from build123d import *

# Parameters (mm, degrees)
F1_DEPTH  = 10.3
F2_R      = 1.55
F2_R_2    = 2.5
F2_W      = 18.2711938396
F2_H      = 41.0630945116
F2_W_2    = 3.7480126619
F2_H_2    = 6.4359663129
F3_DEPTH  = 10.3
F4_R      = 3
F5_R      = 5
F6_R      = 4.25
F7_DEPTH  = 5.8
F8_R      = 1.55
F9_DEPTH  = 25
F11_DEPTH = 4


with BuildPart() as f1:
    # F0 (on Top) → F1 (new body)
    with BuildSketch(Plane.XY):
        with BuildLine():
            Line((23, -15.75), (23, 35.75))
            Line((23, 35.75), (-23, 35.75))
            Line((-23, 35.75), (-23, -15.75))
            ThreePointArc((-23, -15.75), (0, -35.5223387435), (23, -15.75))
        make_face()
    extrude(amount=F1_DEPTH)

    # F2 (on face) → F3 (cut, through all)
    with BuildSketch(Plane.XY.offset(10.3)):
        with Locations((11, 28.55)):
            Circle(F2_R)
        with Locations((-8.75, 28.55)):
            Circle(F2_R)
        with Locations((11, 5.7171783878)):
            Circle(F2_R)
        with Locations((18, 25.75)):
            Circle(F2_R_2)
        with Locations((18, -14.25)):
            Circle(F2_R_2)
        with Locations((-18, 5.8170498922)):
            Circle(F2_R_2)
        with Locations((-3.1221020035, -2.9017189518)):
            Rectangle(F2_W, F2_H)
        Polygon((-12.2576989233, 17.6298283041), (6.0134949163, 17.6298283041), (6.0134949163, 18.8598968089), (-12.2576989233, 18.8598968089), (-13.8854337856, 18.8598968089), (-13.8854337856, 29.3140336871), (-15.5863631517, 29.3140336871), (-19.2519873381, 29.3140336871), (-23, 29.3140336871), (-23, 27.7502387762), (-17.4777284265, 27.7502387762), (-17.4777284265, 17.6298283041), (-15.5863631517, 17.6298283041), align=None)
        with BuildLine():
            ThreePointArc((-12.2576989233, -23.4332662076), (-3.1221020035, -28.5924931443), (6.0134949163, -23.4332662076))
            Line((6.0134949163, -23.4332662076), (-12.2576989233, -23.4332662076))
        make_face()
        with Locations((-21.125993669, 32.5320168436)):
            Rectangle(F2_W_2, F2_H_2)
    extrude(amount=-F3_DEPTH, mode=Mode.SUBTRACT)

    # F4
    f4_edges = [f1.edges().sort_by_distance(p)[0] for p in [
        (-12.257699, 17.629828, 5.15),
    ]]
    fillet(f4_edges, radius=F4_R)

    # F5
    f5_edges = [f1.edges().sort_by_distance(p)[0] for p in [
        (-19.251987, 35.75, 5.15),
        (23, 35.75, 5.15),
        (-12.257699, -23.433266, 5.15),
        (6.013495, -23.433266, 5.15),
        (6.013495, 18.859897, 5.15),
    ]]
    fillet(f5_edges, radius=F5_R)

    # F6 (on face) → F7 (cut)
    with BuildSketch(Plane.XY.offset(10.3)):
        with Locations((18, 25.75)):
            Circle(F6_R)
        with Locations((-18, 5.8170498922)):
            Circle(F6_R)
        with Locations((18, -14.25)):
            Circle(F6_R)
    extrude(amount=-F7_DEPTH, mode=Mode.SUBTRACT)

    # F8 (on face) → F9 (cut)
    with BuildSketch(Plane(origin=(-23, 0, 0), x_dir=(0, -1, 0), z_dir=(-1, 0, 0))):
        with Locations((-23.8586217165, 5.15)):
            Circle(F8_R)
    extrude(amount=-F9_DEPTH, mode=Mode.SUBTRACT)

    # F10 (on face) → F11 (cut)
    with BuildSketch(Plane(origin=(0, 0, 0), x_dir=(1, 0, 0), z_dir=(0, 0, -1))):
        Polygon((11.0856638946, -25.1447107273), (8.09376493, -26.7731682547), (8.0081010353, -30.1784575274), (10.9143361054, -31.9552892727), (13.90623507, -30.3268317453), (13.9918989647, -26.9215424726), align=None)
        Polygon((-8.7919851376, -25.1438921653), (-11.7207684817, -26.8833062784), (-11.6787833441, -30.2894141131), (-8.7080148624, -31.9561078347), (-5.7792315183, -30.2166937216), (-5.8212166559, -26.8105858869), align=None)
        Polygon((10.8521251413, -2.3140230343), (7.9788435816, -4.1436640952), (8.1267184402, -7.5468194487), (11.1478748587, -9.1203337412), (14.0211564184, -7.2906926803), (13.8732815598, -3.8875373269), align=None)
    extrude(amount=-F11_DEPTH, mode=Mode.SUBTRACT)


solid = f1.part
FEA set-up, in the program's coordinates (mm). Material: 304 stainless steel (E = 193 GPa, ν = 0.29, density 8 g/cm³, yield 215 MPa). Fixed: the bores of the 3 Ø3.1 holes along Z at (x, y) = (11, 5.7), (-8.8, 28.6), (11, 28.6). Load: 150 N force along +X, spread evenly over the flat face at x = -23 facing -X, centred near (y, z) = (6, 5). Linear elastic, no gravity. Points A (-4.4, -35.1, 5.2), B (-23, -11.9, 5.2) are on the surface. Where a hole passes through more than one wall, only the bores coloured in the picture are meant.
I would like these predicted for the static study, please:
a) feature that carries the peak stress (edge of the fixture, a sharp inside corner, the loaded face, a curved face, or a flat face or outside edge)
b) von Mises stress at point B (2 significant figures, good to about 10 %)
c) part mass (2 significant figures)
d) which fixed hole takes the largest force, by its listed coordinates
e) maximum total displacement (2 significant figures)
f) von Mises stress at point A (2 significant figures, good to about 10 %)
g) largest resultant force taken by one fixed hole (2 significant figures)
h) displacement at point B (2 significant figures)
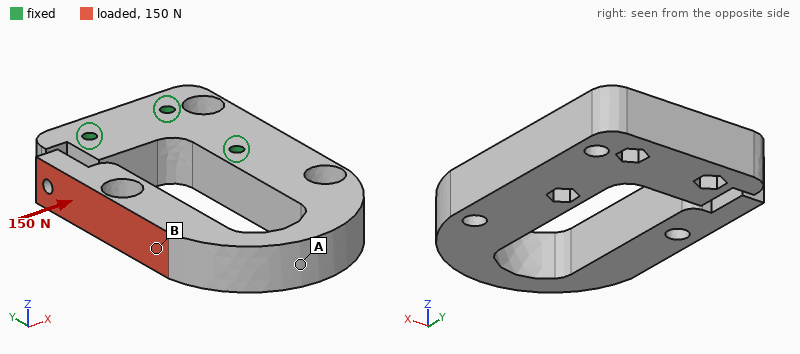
a curved face
13 MPa
160 g
(11, 5.7)
0.20 mm
64 MPa
140 N
0.079 mm
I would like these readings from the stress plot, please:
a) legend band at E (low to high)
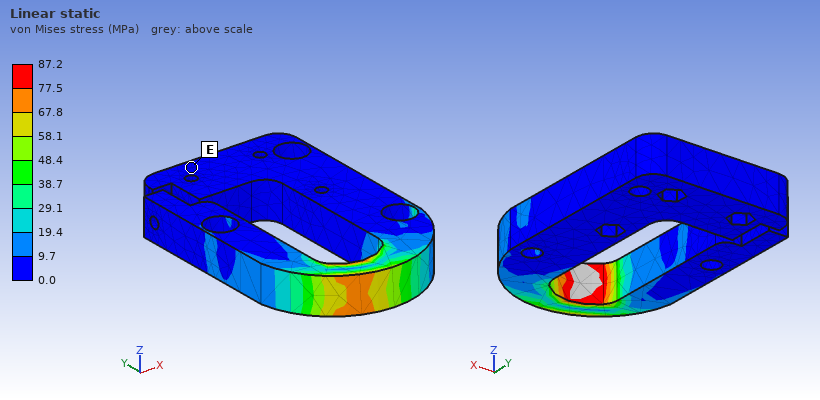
0.0 to 9.7 MPa
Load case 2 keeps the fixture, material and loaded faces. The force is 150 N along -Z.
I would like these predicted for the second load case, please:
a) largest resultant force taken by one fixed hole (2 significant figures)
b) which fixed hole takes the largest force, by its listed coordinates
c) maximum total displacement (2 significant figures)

130 N
(11, 5.7)
0.23 mm
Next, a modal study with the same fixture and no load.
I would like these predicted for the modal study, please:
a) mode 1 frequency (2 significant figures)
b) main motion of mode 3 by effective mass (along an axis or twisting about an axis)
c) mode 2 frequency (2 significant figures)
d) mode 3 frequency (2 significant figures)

930 Hz
along Z
950 Hz
2300 Hz
